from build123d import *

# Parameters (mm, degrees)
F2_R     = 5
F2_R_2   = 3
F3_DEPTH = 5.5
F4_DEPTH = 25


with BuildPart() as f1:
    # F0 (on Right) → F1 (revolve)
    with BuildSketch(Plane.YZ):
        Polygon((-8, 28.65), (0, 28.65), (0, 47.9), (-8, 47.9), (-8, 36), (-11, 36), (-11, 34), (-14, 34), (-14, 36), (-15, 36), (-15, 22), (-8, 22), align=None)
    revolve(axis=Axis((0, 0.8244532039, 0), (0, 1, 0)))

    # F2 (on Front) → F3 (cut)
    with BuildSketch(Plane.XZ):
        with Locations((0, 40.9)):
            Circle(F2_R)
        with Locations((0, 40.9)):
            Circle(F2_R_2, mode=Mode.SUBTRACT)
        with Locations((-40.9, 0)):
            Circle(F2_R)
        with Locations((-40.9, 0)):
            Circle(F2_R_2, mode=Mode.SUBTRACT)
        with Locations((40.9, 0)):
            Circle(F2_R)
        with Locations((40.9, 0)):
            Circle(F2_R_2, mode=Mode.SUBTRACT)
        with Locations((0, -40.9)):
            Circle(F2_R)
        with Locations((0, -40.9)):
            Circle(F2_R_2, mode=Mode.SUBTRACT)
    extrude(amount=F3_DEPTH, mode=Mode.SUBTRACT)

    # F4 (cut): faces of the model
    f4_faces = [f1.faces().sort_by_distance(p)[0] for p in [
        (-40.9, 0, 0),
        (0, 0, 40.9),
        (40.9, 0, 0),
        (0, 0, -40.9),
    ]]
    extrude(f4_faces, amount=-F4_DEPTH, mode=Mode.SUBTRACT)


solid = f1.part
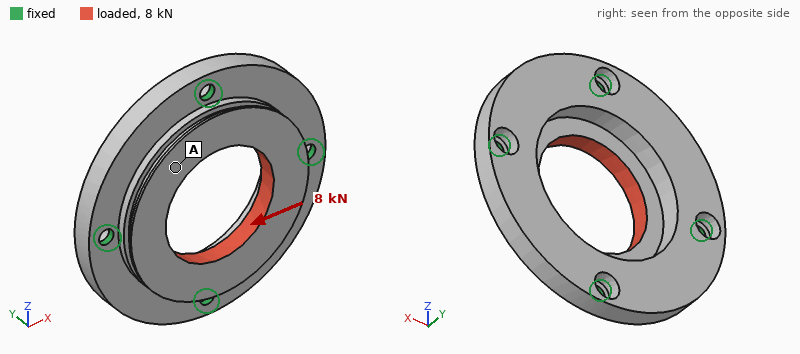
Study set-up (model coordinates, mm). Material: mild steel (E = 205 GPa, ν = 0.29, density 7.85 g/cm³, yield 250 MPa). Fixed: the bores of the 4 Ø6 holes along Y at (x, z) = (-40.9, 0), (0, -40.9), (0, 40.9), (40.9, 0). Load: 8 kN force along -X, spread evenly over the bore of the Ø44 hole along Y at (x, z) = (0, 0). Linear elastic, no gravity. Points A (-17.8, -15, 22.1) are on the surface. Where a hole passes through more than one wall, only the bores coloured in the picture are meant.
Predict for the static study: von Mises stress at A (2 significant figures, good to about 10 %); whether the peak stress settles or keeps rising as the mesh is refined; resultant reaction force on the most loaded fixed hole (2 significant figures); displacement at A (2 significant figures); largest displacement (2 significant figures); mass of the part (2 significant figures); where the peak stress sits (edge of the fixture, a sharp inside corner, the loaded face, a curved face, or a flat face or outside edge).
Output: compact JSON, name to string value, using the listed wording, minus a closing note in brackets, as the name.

{"von Mises stress at A": "8.8 MPa", "whether the peak stress settles or keeps rising as the mesh is refined": "keeps rising", "resultant reaction force on the most loaded fixed hole": "2.1 kN", "displacement at A": "3.5 µm", "largest displacement": "4.3 µm", "mass of the part": "400 g", "where the peak stress sits": "edge of the fixture"}
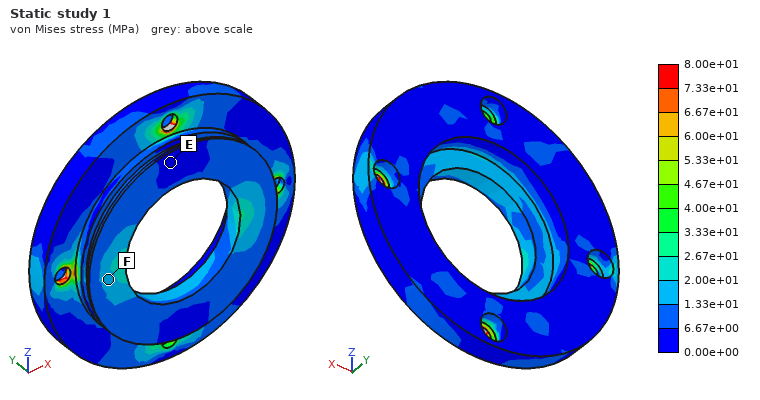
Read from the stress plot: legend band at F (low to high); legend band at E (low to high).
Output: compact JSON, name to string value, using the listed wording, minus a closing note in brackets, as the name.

{"legend band at F": "1.33e+01 to 2.00e+01 MPa", "legend band at E": "0.00e+00 to 6.67e+00 MPa"}
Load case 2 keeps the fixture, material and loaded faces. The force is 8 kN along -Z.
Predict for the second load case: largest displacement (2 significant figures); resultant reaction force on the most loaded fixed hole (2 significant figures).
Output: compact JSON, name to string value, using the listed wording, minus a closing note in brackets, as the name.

{"largest displacement": "4.3 µm", "resultant reaction force on the most loaded fixed hole": "2.1 kN"}
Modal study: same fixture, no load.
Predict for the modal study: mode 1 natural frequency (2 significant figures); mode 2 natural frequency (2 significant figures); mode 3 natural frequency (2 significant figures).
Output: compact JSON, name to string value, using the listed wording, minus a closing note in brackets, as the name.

{"mode 1 natural frequency": "6000 Hz", "mode 2 natural frequency": "8100 Hz", "mode 3 natural frequency": "8100 Hz"}
